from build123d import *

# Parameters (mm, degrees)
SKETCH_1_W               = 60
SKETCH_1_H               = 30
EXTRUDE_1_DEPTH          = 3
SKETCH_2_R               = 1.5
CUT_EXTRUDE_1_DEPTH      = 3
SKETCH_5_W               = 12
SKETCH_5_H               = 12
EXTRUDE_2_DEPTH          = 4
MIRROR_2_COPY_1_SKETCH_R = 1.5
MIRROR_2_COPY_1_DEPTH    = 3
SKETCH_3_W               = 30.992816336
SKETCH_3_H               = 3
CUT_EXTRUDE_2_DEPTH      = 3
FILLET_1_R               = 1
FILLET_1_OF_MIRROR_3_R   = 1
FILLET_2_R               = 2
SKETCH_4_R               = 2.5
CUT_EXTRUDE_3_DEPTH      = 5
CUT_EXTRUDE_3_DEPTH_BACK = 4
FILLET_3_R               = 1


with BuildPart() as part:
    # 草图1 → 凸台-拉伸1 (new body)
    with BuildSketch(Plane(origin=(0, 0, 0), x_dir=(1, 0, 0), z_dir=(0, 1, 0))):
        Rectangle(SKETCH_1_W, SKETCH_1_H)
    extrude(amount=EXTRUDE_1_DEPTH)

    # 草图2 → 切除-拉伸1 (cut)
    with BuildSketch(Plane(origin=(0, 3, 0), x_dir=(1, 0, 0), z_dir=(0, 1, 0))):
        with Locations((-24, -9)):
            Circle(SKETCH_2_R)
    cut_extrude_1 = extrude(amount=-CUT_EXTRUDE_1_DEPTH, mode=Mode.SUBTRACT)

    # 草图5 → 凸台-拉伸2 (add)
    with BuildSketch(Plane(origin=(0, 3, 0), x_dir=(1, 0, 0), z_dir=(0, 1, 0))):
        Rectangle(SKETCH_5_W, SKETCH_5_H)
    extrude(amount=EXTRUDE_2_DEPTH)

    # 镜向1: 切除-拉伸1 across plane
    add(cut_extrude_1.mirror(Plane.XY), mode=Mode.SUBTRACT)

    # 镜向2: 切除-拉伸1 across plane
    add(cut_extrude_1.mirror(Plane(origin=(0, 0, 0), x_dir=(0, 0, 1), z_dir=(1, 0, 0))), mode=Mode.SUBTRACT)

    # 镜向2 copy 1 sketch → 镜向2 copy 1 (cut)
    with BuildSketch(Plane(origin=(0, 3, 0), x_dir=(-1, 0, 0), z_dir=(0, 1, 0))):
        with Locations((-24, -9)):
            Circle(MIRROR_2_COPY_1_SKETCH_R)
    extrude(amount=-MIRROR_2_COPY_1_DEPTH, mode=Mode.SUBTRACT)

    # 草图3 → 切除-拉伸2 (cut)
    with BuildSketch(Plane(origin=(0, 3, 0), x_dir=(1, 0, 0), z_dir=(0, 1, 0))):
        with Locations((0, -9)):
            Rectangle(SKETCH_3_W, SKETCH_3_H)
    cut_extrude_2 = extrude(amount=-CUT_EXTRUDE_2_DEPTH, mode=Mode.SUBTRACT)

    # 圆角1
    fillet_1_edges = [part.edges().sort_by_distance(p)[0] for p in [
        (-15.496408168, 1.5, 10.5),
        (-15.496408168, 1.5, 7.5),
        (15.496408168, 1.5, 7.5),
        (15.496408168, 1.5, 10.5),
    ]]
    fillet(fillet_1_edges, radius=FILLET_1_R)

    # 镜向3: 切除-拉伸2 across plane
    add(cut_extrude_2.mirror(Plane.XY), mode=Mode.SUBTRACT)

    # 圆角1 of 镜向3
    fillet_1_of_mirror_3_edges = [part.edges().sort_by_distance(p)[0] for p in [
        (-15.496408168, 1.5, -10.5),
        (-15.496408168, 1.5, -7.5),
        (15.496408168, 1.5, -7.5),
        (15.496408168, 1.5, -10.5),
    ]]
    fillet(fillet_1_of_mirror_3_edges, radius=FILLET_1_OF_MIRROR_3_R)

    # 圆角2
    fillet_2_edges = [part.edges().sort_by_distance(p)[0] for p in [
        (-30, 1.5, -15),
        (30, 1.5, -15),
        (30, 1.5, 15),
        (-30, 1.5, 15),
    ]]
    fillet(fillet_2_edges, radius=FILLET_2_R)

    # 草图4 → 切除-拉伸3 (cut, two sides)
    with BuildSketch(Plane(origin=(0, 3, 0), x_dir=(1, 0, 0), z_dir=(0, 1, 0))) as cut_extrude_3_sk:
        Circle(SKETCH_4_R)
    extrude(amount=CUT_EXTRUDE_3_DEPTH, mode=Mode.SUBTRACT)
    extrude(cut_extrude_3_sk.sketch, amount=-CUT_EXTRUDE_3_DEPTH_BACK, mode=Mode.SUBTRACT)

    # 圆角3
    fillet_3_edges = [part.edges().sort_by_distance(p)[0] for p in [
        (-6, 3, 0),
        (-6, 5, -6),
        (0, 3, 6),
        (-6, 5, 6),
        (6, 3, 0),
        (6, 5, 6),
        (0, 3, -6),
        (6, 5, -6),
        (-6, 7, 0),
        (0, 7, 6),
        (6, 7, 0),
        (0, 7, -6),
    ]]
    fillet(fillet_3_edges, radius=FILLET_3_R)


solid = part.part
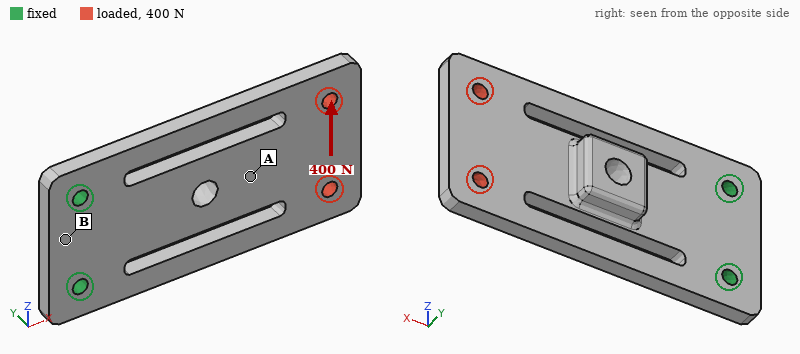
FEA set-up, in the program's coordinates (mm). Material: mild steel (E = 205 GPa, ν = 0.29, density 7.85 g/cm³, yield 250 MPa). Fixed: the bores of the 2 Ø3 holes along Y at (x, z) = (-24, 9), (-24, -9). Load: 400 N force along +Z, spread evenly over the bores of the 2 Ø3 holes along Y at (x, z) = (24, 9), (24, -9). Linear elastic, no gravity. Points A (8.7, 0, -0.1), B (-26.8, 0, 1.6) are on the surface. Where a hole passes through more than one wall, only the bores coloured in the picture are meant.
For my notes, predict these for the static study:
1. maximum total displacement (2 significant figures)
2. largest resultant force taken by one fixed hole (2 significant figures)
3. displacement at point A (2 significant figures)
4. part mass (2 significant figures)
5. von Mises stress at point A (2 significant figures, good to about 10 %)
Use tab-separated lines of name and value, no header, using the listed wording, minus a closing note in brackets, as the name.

maximum total displacement	30 µm
largest resultant force taken by one fixed hole	1.0 kN
displacement at point A	18 µm
part mass	41 g
von Mises stress at point A	23 MPa
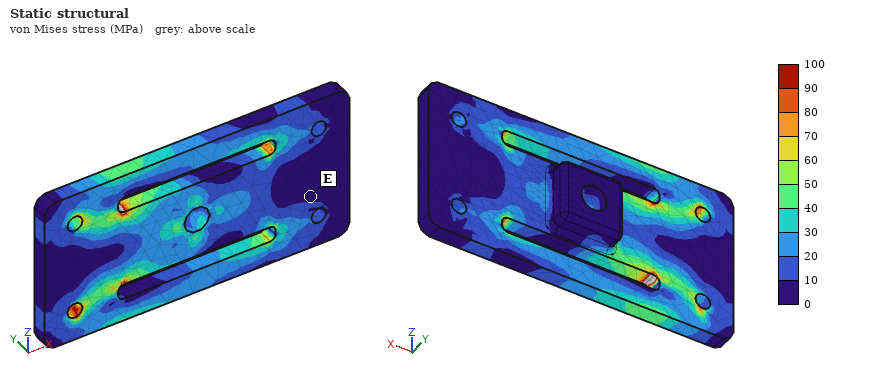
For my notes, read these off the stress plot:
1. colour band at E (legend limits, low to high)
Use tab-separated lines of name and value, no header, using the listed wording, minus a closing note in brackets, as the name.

colour band at E	0 to 10 MPa
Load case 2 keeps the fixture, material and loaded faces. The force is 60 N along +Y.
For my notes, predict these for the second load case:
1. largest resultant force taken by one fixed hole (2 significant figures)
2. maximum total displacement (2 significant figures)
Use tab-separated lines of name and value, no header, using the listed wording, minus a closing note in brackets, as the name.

largest resultant force taken by one fixed hole	31 N
maximum total displacement	0.20 mm
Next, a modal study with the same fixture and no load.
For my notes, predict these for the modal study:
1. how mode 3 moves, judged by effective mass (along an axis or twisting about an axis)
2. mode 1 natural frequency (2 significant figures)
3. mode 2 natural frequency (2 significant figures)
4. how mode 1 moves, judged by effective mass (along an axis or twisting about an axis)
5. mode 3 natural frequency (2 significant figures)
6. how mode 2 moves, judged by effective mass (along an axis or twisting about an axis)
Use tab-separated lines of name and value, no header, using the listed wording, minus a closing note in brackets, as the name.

how mode 3 moves, judged by effective mass	along Z
mode 1 natural frequency	850 Hz
mode 2 natural frequency	3300 Hz
how mode 1 moves, judged by effective mass	along Y
mode 3 natural frequency	5100 Hz
how mode 2 moves, judged by effective mass	twisting about X
